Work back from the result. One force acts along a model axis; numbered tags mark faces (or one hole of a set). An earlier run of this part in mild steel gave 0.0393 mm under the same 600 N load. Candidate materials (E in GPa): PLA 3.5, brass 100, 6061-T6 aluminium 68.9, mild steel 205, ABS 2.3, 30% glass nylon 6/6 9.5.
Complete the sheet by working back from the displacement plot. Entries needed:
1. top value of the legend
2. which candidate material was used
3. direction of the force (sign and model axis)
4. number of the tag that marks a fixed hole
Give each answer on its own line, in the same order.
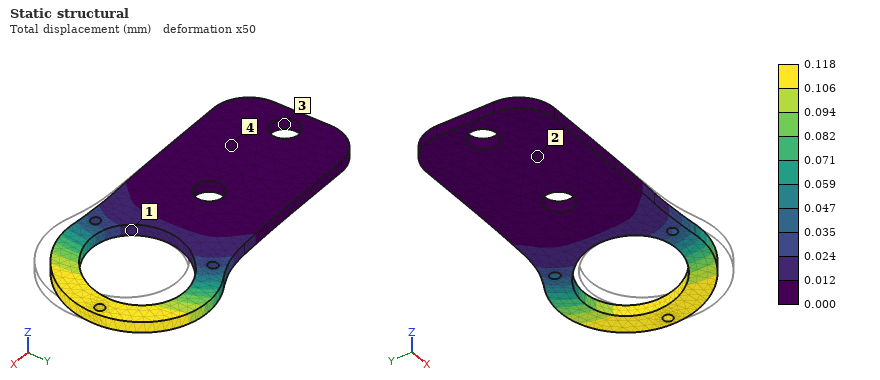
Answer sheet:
0.118 mm
6061-T6 aluminium
+Y
3
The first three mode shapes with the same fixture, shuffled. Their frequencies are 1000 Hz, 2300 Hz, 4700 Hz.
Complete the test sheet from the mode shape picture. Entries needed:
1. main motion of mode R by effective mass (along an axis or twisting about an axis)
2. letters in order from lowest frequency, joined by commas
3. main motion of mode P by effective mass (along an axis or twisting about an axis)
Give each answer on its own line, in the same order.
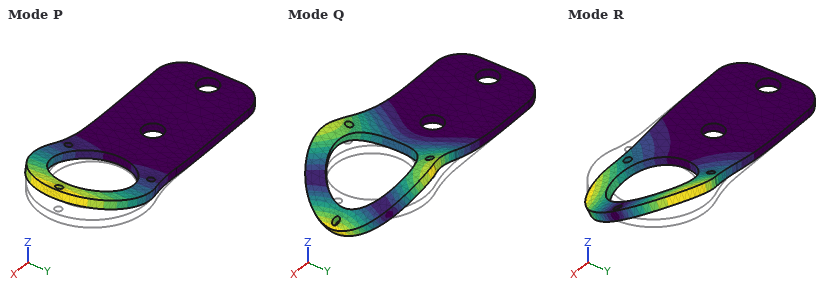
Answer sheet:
twisting about X
P, R, Q
along Z
